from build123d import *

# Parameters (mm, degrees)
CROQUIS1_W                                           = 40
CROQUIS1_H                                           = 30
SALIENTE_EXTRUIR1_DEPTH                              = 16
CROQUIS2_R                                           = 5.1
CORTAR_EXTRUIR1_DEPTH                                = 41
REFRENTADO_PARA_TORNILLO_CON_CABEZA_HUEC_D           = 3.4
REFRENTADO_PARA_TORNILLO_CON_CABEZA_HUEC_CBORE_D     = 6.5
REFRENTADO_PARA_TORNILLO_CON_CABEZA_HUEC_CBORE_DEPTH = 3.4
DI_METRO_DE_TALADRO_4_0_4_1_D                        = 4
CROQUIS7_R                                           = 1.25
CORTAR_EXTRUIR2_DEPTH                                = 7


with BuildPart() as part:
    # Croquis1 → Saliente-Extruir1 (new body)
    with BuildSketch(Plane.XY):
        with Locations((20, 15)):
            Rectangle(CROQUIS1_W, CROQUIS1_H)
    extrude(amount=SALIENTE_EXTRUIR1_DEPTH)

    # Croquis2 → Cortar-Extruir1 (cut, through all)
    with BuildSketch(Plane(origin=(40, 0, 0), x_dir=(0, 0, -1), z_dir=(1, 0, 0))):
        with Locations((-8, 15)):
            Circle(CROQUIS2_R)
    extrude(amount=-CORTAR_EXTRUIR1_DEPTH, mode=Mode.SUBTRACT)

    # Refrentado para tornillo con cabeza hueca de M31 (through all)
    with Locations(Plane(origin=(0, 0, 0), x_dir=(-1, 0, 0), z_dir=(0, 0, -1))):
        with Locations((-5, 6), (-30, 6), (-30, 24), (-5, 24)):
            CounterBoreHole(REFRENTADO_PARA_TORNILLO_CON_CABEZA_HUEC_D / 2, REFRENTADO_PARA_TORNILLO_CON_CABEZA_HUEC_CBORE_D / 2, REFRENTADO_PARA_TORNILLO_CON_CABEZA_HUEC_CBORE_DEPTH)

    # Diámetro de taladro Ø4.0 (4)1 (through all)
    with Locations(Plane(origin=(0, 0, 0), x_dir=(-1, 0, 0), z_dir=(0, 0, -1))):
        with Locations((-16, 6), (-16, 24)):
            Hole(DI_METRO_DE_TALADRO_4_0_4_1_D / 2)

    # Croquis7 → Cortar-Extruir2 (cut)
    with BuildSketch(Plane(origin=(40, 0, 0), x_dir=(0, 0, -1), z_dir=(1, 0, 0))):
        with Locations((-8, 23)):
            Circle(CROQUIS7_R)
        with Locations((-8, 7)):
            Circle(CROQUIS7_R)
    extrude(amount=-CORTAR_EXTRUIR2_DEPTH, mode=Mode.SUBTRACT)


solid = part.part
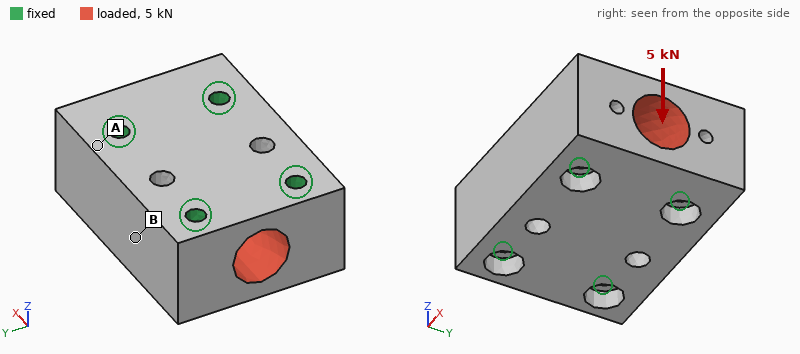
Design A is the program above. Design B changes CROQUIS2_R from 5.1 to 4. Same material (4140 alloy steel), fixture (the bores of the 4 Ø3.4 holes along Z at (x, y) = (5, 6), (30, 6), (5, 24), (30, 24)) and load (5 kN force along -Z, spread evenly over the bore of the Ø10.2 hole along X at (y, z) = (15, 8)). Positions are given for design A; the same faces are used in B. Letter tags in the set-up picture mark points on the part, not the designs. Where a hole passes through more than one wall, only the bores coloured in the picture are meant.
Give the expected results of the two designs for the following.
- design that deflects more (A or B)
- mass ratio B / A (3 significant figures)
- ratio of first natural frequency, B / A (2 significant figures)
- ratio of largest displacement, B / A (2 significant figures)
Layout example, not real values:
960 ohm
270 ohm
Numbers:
A
1.09
0.99
0.86
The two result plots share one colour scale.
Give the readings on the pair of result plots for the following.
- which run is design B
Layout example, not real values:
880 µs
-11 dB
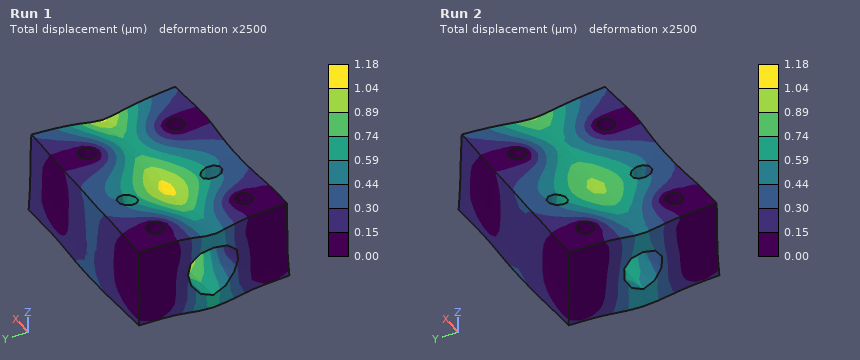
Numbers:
Run 2
